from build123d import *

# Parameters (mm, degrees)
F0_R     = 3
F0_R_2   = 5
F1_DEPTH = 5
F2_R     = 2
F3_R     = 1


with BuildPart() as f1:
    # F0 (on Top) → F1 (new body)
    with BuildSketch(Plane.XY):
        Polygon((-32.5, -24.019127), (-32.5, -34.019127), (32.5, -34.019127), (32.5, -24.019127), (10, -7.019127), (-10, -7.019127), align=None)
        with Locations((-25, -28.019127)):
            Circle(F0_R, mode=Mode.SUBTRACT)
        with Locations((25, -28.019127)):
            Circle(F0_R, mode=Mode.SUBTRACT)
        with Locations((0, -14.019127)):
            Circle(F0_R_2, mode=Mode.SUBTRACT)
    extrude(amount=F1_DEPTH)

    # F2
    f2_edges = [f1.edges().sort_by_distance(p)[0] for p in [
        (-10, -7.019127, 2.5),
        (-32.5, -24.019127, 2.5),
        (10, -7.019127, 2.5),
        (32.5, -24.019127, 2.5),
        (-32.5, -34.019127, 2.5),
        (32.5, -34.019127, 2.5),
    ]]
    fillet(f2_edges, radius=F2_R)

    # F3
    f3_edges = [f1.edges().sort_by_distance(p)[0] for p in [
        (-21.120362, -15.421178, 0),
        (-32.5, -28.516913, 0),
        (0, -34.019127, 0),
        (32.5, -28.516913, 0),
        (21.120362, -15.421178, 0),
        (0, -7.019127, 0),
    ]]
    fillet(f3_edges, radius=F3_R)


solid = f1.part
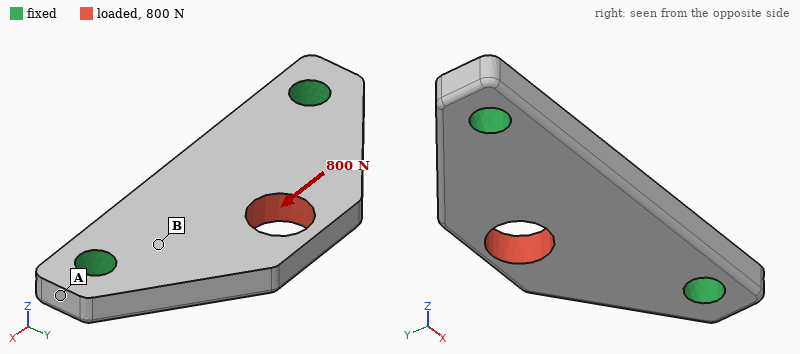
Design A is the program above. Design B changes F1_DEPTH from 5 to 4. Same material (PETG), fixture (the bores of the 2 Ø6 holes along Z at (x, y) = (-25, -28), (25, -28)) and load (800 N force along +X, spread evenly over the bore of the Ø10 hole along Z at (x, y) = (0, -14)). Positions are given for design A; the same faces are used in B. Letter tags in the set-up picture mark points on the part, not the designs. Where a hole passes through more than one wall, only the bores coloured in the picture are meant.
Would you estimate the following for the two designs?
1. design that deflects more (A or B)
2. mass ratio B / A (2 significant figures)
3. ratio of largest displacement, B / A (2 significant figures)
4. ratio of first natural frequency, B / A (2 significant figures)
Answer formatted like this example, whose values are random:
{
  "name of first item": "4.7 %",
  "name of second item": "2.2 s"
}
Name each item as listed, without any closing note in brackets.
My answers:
{
  "design that deflects more": "B",
  "mass ratio B / A": "0.80",
  "ratio of largest displacement, B / A": "1.3",
  "ratio of first natural frequency, B / A": "0.83"
}
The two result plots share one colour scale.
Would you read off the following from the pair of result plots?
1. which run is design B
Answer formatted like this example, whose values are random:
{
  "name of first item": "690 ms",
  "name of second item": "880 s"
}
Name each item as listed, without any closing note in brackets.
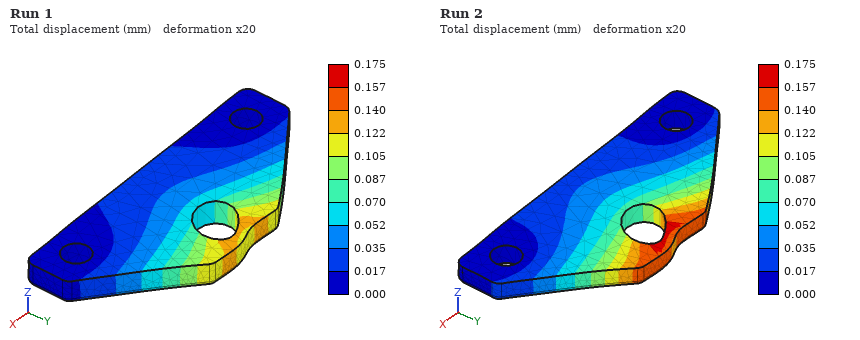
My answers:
{
  "which run is design B": "Run 2"
}
